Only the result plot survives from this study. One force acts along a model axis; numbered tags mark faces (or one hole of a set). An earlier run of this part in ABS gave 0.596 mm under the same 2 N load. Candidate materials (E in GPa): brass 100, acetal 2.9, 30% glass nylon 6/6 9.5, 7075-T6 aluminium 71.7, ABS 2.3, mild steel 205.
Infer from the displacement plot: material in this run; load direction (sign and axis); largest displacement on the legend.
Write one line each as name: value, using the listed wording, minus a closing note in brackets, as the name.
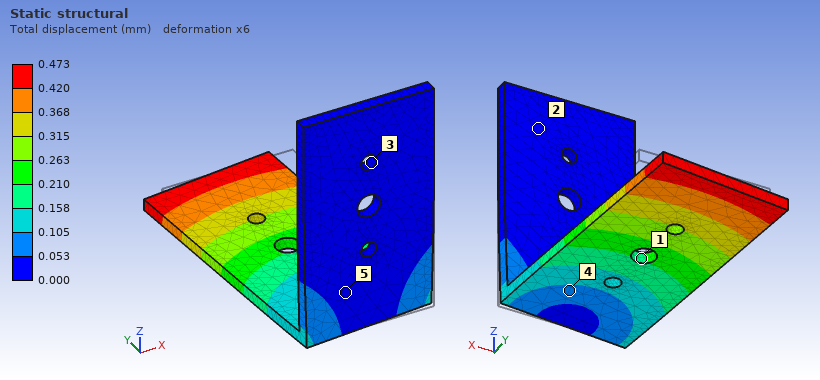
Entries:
material in this run: acetal
load direction: -X
largest displacement on the legend: 0.473 mm
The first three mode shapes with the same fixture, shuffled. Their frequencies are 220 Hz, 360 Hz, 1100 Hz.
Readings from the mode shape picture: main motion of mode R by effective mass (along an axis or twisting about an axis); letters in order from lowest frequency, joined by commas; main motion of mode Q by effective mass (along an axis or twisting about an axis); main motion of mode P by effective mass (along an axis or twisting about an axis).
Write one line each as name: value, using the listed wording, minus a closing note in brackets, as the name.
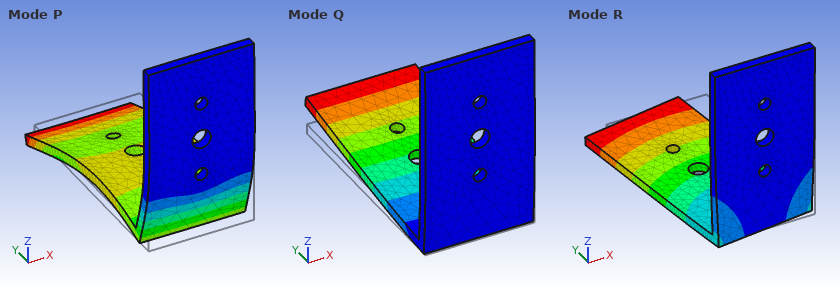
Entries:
main motion of mode R by effective mass: along X
letters in order from lowest frequency, joined by commas: Q, R, P
main motion of mode Q by effective mass: along Z
main motion of mode P by effective mass: along Y
